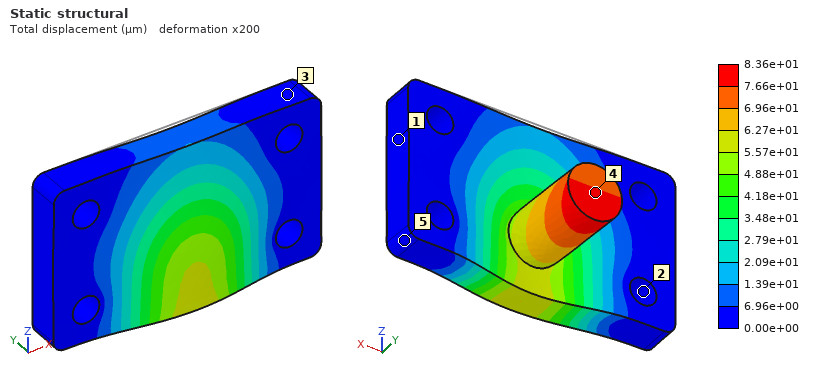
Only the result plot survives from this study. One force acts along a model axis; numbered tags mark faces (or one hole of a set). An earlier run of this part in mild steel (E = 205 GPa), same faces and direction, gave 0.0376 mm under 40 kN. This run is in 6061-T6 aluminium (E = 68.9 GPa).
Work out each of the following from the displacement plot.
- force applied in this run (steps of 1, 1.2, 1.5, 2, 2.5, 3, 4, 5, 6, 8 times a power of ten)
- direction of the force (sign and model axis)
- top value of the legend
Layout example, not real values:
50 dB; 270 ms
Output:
30 kN; -Y; 8.36e+01 µm
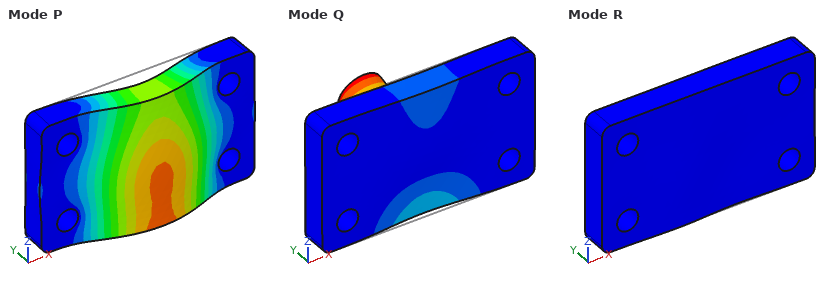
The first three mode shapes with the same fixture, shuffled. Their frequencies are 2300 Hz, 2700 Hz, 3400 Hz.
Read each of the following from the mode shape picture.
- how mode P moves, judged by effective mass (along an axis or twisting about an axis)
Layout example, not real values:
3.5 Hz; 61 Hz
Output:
along Y
